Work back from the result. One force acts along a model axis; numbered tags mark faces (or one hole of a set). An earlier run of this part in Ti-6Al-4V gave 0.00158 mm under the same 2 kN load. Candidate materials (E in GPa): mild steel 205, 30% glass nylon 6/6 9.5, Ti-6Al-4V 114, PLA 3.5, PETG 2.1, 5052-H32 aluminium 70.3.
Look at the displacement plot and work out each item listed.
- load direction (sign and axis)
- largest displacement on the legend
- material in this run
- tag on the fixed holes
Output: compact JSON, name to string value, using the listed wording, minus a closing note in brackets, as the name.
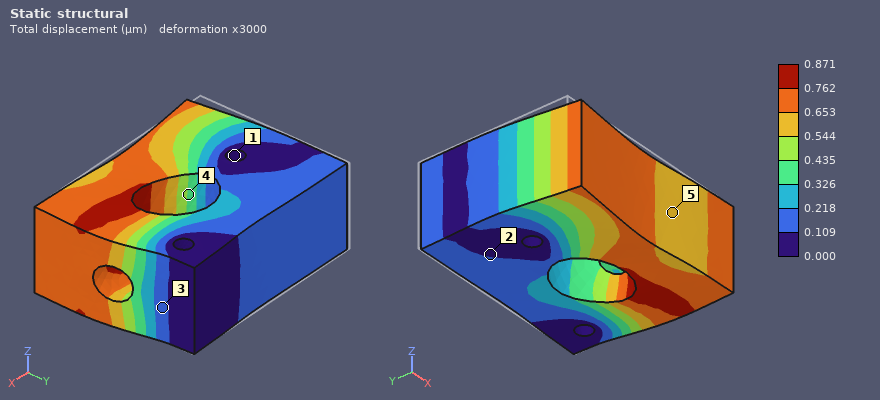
{"load direction": "+X", "largest displacement on the legend": "0.871 µm", "material in this run": "mild steel", "tag on the fixed holes": "1"}
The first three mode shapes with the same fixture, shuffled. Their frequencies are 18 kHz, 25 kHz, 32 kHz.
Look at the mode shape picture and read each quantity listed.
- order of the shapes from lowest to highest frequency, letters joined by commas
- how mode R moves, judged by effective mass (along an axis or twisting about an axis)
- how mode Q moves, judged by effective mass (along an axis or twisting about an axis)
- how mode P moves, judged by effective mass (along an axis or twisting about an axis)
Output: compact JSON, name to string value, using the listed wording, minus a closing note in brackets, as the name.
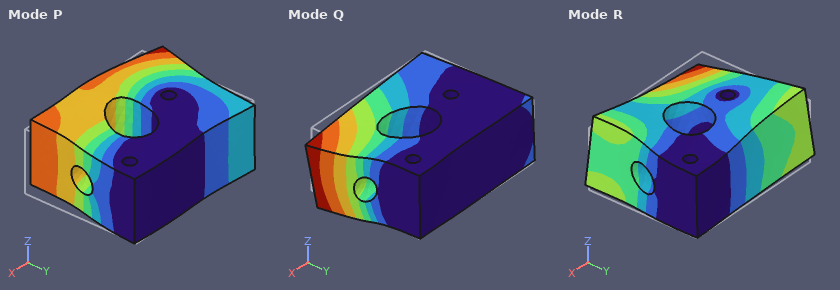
{"order of the shapes from lowest to highest frequency, letters joined by commas": "Q, P, R", "how mode R moves, judged by effective mass": "twisting about X", "how mode Q moves, judged by effective mass": "along Z", "how mode P moves, judged by effective mass": "along X"}
